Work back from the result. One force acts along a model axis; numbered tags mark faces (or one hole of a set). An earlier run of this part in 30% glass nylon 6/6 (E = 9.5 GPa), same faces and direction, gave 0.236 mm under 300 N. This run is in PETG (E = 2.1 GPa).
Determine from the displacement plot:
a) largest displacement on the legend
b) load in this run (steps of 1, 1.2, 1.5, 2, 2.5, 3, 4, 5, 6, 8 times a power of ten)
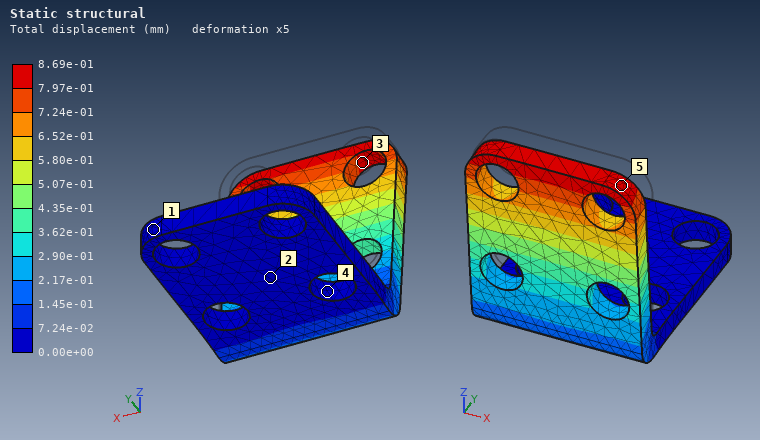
8.69e-01 mm
250 N
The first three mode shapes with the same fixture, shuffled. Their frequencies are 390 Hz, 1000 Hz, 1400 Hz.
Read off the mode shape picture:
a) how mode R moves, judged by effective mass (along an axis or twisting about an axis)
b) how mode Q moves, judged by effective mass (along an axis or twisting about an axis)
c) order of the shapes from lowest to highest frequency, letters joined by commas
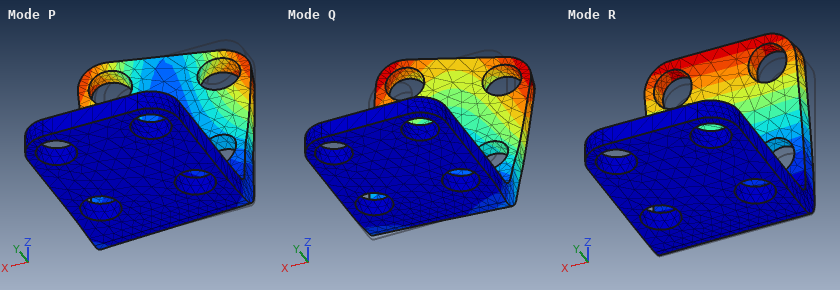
along Y
along X
R, Q, P
